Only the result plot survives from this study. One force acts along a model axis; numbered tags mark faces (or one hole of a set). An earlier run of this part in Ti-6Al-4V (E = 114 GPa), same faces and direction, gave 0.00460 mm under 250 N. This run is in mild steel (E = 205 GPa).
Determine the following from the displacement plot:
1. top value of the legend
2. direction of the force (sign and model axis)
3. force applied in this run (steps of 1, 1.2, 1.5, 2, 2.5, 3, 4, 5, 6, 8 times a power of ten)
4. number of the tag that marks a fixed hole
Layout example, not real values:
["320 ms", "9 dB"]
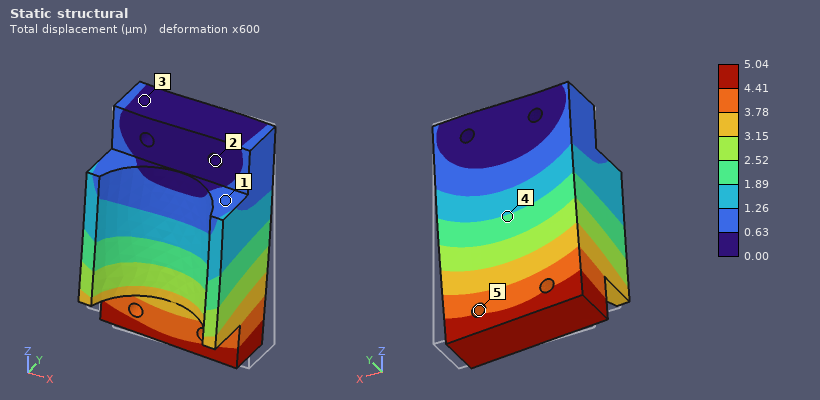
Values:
["5.04 µm", "-X", "500 N", "2"]
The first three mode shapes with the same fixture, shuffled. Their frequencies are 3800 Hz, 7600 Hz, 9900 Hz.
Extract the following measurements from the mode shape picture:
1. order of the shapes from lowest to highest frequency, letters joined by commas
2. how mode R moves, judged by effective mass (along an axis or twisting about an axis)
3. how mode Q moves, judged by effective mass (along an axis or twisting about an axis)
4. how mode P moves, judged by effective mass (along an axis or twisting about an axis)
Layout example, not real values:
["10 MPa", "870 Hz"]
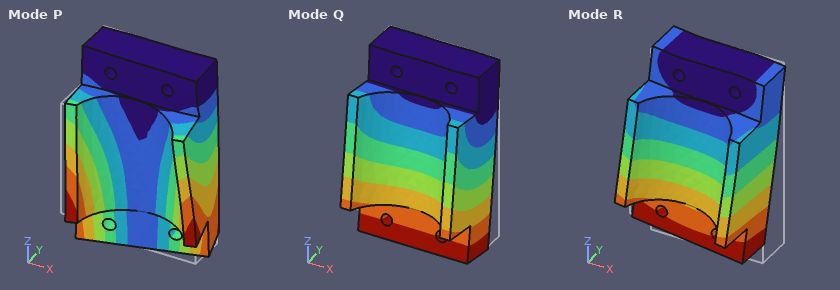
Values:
["Q, R, P", "along X", "along Y", "twisting about Z"]
